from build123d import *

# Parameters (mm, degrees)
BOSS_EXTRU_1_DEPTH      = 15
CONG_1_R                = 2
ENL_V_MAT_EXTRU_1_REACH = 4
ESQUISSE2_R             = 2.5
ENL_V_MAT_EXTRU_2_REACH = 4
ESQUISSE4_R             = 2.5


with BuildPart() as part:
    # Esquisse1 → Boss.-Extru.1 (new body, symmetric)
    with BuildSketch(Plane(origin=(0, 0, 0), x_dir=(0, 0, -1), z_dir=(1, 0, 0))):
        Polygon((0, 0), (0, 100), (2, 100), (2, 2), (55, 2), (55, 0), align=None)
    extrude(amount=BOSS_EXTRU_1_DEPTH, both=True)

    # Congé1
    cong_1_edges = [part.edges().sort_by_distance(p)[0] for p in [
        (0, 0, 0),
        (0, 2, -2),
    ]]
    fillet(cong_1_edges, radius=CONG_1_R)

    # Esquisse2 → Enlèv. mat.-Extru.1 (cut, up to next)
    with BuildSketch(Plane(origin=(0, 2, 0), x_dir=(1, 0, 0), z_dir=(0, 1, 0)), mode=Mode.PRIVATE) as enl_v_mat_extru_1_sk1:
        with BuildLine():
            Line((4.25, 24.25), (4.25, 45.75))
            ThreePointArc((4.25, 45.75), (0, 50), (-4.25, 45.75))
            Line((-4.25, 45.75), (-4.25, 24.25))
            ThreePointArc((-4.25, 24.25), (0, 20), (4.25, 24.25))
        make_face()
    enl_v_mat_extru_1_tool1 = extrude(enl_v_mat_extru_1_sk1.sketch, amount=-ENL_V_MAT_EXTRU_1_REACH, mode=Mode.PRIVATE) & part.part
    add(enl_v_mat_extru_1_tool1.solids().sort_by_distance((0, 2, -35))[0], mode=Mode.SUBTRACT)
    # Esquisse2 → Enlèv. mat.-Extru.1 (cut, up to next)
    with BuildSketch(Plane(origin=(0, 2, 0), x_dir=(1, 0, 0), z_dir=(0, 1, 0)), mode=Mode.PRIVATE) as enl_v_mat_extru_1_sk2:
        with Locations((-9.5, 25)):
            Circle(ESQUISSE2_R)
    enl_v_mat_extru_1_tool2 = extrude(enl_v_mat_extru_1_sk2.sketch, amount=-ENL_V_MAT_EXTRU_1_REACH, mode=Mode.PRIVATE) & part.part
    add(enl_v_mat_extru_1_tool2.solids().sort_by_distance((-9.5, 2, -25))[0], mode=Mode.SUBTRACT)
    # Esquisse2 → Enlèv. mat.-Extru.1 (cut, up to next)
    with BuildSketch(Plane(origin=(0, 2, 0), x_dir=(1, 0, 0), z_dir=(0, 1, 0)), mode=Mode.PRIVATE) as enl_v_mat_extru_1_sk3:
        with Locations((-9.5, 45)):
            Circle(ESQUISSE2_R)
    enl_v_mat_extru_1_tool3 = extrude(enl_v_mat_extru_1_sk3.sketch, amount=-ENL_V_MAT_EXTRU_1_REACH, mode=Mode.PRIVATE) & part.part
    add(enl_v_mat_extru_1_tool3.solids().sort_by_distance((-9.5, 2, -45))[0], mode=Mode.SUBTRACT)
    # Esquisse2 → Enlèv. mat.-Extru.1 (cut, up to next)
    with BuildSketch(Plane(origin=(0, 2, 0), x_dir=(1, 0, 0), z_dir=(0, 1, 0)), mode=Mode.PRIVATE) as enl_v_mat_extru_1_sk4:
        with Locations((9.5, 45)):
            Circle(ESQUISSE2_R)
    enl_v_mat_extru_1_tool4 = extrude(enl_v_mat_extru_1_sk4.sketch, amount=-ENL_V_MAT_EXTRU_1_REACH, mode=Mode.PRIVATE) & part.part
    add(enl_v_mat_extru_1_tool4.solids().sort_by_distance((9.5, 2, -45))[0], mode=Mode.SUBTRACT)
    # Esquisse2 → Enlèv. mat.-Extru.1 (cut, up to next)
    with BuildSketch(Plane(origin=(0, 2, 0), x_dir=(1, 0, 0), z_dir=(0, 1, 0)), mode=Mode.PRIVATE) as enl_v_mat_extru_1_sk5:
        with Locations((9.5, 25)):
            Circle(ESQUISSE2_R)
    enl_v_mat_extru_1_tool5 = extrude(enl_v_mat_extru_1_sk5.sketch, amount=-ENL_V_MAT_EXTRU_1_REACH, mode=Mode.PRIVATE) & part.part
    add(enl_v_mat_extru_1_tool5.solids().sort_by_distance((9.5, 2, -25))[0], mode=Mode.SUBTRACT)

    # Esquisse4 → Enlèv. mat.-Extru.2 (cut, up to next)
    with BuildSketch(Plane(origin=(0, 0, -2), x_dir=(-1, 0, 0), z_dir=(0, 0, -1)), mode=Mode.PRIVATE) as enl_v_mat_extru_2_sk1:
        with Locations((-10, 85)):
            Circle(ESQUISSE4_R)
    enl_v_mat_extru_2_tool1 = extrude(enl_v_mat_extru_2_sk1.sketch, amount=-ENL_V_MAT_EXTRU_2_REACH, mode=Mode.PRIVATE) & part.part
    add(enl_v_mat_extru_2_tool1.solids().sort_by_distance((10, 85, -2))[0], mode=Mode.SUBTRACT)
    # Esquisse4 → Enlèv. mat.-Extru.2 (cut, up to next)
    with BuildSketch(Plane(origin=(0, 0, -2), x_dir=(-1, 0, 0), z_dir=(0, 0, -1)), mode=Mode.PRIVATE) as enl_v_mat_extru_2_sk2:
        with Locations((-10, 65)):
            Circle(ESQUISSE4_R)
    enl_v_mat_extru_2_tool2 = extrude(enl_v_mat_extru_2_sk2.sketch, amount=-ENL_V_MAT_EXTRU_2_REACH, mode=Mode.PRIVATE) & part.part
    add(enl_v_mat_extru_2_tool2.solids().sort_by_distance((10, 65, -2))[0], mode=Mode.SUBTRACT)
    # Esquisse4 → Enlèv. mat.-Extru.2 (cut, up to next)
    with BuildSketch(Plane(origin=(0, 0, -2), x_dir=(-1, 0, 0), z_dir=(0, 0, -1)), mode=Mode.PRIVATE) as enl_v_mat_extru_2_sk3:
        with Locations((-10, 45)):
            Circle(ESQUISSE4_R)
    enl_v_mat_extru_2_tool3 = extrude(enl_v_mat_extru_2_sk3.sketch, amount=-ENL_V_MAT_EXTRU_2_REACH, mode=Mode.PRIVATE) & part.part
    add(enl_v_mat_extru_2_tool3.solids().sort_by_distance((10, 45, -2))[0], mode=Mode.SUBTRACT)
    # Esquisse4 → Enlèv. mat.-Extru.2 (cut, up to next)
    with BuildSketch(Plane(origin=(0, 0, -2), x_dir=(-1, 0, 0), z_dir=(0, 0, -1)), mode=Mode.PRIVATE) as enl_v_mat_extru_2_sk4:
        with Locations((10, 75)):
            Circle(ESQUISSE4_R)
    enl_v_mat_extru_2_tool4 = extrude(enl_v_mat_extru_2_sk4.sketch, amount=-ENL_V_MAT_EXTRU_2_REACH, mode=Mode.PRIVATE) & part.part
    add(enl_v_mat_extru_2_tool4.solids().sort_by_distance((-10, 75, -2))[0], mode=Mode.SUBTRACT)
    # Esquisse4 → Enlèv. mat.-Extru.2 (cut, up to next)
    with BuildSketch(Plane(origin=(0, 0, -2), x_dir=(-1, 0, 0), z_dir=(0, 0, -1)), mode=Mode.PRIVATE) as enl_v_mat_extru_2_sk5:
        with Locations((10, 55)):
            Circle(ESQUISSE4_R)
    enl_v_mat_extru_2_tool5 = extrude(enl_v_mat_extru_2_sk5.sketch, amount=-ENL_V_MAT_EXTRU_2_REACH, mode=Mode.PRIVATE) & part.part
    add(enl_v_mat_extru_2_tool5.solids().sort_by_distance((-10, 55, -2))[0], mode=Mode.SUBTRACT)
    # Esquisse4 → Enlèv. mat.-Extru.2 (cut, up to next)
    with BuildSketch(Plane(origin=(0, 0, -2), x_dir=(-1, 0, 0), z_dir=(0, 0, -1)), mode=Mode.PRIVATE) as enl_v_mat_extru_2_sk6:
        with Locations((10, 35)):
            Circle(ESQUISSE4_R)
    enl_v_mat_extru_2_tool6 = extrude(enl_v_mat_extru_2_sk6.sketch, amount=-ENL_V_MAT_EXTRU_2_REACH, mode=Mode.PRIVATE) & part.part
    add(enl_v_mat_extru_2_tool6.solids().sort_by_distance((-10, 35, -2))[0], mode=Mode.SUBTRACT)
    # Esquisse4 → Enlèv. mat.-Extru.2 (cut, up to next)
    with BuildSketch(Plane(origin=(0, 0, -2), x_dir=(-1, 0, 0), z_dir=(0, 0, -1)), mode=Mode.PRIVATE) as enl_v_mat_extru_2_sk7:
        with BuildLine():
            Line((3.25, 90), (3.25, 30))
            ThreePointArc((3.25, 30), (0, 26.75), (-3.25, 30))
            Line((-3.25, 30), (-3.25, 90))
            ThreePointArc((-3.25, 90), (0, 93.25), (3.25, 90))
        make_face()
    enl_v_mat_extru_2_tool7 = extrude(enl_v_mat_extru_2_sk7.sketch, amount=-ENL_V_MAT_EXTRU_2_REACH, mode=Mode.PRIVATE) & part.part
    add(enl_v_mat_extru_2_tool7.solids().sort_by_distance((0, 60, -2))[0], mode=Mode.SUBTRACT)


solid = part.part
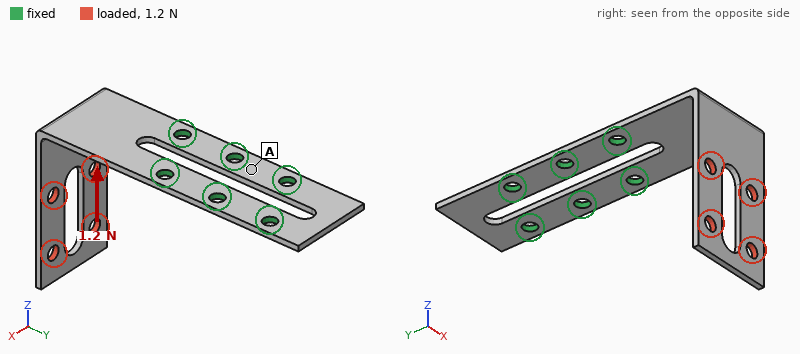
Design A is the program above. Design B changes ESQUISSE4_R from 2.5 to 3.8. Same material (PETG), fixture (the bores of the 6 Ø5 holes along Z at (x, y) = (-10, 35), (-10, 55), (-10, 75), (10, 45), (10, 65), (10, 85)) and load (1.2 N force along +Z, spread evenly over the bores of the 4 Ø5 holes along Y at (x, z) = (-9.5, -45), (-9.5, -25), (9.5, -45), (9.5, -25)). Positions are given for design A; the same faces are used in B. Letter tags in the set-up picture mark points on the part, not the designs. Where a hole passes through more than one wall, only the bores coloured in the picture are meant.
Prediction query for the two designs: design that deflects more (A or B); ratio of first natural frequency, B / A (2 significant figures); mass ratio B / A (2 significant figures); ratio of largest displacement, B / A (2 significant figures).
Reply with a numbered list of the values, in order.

1. A
2. 1.0
3. 0.96
4. 0.89
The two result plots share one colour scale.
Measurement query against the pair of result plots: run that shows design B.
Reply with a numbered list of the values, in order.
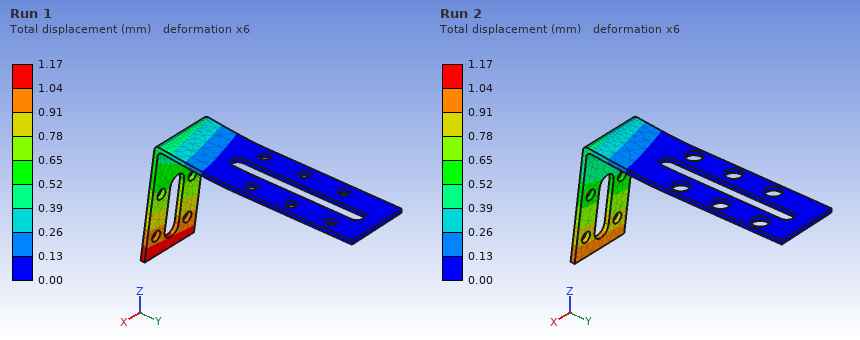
1. Run 2
